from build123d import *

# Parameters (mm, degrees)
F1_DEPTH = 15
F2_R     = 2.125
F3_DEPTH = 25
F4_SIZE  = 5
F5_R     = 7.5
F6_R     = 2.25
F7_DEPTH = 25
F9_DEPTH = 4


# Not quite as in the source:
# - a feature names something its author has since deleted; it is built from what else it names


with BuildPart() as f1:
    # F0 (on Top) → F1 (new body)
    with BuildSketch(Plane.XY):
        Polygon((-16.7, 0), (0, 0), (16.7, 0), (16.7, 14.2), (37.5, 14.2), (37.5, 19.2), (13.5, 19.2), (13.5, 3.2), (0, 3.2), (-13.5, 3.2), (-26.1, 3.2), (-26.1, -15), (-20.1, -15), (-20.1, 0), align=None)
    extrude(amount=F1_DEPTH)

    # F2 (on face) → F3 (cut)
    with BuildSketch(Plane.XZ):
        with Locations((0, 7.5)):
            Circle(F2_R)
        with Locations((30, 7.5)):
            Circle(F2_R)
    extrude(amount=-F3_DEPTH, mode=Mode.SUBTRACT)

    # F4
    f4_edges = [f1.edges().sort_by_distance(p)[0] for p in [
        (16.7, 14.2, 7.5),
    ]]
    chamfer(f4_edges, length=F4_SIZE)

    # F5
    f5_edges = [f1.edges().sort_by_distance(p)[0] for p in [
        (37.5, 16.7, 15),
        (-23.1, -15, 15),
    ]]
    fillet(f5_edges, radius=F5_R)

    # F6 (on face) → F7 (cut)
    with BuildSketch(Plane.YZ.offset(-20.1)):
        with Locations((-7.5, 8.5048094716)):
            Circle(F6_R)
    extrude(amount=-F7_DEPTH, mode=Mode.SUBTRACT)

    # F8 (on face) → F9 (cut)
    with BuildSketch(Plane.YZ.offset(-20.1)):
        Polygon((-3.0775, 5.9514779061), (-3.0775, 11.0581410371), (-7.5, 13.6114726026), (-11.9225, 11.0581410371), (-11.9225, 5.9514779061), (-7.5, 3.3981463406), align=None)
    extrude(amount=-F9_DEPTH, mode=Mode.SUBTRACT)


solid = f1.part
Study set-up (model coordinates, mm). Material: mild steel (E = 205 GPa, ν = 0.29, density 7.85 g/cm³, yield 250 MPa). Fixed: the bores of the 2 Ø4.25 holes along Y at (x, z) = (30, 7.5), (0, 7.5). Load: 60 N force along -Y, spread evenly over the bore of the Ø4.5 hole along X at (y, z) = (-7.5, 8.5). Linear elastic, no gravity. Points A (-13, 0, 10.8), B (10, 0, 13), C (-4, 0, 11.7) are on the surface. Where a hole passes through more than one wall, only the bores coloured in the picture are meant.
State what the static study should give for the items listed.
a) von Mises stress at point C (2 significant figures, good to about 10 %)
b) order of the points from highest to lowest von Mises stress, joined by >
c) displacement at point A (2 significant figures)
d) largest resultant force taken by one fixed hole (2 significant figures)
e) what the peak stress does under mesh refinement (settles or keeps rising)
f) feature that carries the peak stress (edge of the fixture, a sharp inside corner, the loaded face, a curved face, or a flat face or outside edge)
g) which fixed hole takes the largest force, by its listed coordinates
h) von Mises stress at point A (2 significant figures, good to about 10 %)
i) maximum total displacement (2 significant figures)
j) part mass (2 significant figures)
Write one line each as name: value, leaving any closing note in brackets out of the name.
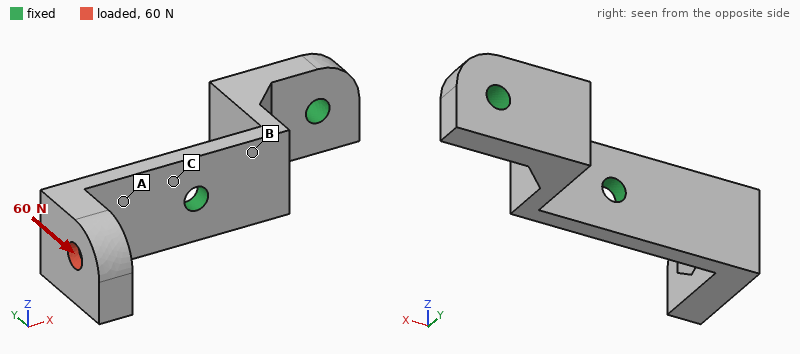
von Mises stress at point C: 43 MPa
order of the points from highest to lowest von Mises stress, joined by >: C > A > B
displacement at point A: 11 µm
largest resultant force taken by one fixed hole: 69 N
what the peak stress does under mesh refinement: keeps rising
feature that carries the peak stress: edge of the fixture
which fixed hole takes the largest force, by its listed coordinates: (0, 7.5)
von Mises stress at point A: 27 MPa
maximum total displacement: 49 µm
part mass: 42 g
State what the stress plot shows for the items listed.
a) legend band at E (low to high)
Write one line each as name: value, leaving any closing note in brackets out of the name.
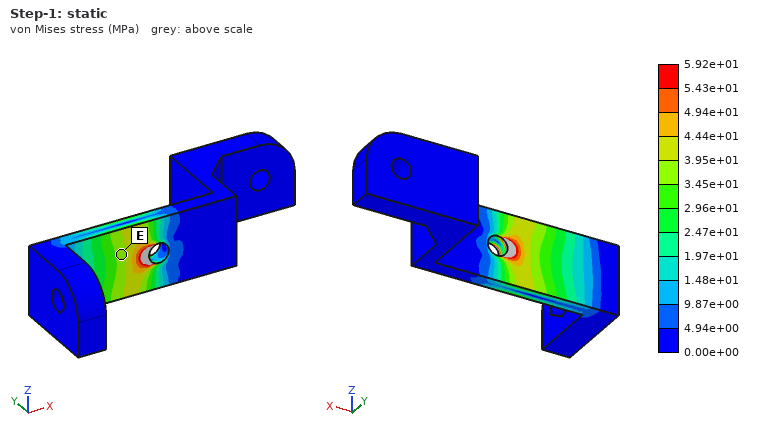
legend band at E: 3.45e+01 to 3.95e+01 MPa
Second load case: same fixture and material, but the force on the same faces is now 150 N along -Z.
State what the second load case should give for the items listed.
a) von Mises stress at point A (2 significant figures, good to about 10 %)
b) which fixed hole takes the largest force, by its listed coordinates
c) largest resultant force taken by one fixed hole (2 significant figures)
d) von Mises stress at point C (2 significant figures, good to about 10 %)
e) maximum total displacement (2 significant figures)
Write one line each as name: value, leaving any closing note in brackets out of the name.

von Mises stress at point A: 53 MPa
which fixed hole takes the largest force, by its listed coordinates: (0, 7.5)
largest resultant force taken by one fixed hole: 180 N
von Mises stress at point C: 39 MPa
maximum total displacement: 47 µm
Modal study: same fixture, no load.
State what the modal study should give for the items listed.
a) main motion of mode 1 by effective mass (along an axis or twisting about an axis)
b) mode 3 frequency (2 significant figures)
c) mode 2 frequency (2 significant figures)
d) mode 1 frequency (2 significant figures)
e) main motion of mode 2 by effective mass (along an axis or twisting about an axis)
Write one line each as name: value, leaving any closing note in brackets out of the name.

main motion of mode 1 by effective mass: along Y
mode 3 frequency: 7800 Hz
mode 2 frequency: 3700 Hz
mode 1 frequency: 2000 Hz
main motion of mode 2 by effective mass: along Z
